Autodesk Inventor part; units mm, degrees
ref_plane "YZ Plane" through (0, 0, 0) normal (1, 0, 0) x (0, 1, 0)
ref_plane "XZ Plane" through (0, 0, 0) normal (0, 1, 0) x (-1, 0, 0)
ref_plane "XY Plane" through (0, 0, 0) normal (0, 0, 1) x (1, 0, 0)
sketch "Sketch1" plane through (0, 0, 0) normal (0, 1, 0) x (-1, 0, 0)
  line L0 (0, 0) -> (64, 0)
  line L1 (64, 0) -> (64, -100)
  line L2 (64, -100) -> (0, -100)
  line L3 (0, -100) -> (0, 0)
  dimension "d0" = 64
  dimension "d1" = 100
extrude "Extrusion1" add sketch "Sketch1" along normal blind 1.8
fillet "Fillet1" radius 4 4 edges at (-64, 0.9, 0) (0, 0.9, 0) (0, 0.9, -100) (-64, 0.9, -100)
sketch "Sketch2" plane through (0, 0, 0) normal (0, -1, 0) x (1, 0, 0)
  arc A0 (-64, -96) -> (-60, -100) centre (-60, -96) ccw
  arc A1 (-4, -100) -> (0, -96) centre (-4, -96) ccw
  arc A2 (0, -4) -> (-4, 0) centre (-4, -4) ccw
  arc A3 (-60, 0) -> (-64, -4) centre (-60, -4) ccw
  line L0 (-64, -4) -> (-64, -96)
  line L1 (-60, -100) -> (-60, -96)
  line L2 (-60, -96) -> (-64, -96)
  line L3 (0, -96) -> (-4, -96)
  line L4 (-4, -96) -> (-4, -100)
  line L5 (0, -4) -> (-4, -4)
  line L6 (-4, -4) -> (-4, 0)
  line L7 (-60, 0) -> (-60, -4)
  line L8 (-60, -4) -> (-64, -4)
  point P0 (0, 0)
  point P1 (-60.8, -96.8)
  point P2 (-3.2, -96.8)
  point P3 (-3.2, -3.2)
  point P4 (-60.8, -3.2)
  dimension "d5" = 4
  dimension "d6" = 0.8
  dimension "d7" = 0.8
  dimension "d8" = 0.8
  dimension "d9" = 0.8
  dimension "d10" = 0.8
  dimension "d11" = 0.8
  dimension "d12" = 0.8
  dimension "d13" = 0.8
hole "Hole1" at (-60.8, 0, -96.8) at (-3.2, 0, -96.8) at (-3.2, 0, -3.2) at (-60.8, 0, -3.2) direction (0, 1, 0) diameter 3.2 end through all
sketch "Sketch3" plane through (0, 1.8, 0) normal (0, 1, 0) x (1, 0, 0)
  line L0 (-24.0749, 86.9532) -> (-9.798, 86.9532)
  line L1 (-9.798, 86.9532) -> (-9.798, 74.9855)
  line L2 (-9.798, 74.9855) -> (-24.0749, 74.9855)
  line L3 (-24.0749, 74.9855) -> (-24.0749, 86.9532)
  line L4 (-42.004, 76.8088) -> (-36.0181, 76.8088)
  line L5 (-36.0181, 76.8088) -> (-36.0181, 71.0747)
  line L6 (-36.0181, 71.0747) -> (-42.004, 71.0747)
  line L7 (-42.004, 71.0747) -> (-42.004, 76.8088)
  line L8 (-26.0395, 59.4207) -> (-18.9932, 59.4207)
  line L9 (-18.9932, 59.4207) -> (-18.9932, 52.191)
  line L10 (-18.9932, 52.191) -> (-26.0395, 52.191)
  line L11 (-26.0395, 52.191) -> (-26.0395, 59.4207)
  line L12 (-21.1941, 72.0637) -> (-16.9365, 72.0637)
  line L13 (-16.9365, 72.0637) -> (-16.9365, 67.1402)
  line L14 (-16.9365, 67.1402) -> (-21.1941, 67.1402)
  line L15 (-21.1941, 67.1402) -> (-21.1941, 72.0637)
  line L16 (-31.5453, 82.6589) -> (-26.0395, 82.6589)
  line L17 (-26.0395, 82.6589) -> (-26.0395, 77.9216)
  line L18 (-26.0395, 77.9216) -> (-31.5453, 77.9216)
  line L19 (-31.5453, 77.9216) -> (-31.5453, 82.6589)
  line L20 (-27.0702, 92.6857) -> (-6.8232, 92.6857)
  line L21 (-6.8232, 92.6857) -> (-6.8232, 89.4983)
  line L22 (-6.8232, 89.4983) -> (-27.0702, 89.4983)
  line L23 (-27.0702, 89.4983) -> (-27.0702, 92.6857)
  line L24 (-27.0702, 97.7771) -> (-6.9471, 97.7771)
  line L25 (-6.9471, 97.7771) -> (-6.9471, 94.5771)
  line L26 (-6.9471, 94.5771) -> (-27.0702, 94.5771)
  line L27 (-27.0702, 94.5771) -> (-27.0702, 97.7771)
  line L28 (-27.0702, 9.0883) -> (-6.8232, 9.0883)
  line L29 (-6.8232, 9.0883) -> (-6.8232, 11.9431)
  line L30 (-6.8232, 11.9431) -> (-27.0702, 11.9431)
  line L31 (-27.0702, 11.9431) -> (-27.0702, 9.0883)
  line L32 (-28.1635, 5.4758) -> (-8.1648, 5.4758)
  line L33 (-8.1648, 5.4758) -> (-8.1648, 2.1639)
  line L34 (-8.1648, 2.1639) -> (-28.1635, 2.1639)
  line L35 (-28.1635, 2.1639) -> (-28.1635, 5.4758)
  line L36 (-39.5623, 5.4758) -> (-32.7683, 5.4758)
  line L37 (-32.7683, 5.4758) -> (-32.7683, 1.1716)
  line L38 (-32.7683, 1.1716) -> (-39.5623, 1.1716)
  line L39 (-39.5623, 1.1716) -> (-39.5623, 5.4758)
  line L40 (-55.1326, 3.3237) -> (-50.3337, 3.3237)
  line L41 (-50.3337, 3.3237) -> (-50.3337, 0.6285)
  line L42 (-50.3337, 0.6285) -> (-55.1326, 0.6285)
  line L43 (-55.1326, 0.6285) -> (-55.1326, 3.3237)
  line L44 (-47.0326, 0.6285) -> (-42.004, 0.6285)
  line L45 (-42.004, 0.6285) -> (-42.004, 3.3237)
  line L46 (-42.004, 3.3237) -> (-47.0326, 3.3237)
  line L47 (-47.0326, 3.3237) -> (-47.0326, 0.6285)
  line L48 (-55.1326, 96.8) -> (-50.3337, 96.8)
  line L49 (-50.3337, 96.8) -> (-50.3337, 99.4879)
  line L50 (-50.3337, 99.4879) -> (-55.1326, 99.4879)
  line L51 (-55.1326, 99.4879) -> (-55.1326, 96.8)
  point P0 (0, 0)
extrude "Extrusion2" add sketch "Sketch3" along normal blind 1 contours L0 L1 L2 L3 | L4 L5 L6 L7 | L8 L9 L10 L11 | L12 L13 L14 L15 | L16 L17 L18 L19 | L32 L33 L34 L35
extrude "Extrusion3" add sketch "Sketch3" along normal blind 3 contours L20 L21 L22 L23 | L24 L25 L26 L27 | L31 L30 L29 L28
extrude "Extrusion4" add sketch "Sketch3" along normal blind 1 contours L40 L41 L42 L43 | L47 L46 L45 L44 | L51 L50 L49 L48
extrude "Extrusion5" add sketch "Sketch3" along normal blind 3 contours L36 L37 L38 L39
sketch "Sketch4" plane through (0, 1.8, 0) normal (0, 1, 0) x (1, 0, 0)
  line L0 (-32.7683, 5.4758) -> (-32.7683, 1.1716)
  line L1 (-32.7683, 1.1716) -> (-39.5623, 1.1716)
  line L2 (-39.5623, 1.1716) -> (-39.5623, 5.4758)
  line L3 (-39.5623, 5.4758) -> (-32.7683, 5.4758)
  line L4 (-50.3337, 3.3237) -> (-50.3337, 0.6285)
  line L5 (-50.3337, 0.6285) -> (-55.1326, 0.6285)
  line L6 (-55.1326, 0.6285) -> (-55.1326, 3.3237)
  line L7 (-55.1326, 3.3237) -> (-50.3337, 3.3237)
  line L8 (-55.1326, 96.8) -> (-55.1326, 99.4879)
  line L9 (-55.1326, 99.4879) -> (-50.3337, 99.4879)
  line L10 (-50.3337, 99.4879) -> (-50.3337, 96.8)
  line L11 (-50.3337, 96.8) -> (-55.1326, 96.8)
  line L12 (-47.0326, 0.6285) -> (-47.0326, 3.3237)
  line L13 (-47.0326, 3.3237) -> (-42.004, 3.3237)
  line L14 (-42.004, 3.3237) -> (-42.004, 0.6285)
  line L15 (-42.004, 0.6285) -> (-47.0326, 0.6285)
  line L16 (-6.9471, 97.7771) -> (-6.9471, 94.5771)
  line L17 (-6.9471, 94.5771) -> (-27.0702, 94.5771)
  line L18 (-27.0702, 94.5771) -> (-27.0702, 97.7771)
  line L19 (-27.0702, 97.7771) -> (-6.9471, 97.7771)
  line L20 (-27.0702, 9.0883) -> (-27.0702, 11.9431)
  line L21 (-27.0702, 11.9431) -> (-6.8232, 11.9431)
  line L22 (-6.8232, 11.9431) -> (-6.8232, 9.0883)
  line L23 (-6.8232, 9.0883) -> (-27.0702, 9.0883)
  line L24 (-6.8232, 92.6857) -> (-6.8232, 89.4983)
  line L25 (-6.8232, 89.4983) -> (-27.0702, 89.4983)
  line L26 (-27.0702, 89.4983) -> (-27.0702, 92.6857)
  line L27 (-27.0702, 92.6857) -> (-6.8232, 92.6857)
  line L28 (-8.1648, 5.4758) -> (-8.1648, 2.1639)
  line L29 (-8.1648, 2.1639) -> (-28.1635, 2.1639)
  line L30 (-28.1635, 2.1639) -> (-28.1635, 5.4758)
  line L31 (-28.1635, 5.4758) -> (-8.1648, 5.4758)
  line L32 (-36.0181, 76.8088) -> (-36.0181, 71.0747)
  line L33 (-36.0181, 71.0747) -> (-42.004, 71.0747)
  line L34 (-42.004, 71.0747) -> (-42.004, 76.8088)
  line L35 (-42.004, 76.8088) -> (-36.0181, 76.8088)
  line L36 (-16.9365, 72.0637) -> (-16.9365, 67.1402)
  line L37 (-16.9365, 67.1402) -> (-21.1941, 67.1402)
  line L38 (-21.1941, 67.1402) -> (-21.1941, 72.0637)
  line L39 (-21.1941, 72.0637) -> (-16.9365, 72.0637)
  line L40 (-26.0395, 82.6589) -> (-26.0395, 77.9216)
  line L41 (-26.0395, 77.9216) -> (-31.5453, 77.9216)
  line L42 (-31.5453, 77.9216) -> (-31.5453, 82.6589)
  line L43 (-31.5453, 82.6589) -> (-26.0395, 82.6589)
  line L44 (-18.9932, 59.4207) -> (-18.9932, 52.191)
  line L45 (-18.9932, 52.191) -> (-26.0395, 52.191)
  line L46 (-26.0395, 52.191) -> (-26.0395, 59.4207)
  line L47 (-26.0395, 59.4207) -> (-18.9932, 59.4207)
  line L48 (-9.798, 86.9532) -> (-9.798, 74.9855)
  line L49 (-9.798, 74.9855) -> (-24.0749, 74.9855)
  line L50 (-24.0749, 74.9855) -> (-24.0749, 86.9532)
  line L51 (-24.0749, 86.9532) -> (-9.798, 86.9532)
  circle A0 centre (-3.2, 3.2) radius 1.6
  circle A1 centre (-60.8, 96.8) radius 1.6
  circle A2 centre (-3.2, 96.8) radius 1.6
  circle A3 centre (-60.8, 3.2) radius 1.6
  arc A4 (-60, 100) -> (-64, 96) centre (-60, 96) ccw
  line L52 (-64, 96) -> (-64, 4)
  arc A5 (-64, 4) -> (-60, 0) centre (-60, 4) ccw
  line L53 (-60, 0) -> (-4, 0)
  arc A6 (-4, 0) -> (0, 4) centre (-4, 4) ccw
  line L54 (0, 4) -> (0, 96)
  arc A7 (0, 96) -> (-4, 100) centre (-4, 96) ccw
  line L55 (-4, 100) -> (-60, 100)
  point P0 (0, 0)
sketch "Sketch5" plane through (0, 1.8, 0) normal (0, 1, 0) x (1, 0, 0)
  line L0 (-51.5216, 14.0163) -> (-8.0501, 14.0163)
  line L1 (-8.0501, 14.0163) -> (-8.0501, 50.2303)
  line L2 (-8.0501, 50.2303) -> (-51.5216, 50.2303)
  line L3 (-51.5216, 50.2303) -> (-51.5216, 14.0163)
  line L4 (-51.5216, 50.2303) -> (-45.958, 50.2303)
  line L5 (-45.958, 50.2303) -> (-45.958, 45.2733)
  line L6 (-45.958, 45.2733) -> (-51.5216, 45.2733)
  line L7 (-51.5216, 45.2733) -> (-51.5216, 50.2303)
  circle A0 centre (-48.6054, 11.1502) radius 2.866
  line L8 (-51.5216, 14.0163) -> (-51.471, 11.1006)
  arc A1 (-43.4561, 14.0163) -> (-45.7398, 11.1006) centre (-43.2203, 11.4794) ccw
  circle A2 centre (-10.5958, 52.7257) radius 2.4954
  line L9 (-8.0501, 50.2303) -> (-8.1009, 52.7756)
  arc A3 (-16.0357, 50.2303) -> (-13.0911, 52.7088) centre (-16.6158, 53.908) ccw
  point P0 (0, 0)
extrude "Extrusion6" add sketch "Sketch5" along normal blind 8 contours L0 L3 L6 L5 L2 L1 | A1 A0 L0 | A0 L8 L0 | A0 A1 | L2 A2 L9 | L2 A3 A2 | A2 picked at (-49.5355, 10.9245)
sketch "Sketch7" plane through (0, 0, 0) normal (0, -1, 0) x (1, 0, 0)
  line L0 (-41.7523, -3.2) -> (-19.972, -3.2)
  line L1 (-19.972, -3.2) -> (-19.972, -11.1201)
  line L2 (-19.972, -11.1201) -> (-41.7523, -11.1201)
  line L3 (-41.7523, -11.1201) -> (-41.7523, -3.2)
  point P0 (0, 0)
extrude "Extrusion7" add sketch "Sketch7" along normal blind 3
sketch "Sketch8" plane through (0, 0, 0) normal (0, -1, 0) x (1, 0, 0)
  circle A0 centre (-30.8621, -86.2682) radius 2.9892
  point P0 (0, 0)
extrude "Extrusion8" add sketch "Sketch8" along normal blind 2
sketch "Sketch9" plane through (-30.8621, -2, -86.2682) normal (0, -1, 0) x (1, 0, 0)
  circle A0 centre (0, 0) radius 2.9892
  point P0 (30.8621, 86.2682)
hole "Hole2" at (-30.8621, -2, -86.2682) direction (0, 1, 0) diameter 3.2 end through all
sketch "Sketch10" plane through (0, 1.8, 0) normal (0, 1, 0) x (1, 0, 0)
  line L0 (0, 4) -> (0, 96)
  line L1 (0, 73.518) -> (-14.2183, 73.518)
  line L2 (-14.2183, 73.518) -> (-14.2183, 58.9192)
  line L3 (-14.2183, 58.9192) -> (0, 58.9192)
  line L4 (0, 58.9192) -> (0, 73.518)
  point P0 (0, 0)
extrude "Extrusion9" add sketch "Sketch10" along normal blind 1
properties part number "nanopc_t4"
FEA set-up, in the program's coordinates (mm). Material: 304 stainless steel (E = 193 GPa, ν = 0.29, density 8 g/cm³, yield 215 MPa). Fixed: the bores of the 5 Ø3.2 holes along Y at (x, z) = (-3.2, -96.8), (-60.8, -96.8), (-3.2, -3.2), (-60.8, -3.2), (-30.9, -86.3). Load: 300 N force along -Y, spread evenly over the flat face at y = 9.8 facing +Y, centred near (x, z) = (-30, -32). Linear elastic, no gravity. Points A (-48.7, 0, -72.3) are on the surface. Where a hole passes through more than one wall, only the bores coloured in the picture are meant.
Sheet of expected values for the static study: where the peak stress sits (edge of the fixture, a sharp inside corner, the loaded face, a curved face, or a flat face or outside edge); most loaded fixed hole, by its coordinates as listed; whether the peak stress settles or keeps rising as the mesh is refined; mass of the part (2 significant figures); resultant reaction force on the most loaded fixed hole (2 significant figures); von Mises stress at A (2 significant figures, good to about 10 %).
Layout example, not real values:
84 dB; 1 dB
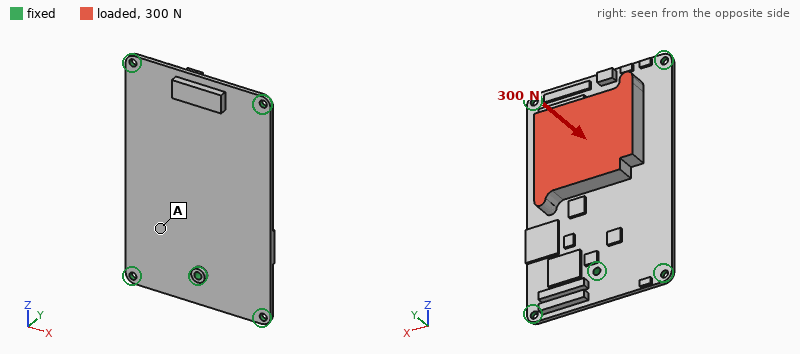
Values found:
edge of the fixture; (-3.2, -3.2); keeps rising; 210 g; 140 N; 7.8 MPa
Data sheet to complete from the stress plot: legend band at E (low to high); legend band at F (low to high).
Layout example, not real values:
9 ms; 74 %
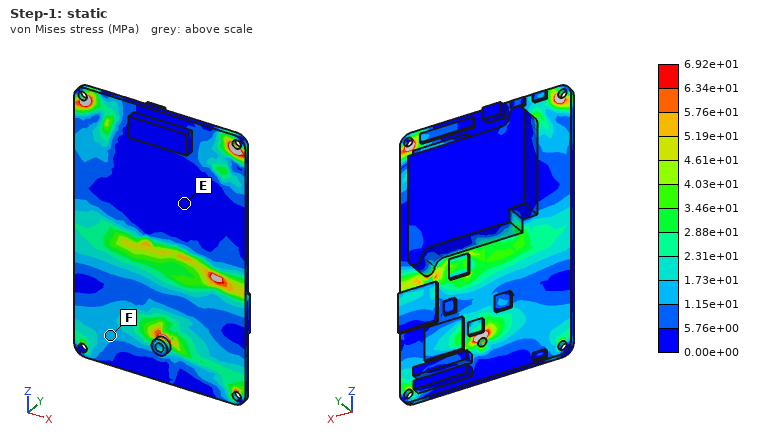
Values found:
0.00e+00 to 5.76e+00 MPa; 1.15e+01 to 1.73e+01 MPa
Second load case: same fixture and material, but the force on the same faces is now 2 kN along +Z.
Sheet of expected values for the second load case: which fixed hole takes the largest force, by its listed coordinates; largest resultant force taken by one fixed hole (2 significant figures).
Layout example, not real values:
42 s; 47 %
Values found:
(-30.9, -86.3); 640 N
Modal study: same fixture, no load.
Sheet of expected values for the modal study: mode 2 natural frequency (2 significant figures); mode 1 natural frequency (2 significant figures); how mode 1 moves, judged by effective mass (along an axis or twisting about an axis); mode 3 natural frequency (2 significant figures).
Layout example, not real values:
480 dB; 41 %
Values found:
2400 Hz; 1000 Hz; along Y; 3100 Hz
